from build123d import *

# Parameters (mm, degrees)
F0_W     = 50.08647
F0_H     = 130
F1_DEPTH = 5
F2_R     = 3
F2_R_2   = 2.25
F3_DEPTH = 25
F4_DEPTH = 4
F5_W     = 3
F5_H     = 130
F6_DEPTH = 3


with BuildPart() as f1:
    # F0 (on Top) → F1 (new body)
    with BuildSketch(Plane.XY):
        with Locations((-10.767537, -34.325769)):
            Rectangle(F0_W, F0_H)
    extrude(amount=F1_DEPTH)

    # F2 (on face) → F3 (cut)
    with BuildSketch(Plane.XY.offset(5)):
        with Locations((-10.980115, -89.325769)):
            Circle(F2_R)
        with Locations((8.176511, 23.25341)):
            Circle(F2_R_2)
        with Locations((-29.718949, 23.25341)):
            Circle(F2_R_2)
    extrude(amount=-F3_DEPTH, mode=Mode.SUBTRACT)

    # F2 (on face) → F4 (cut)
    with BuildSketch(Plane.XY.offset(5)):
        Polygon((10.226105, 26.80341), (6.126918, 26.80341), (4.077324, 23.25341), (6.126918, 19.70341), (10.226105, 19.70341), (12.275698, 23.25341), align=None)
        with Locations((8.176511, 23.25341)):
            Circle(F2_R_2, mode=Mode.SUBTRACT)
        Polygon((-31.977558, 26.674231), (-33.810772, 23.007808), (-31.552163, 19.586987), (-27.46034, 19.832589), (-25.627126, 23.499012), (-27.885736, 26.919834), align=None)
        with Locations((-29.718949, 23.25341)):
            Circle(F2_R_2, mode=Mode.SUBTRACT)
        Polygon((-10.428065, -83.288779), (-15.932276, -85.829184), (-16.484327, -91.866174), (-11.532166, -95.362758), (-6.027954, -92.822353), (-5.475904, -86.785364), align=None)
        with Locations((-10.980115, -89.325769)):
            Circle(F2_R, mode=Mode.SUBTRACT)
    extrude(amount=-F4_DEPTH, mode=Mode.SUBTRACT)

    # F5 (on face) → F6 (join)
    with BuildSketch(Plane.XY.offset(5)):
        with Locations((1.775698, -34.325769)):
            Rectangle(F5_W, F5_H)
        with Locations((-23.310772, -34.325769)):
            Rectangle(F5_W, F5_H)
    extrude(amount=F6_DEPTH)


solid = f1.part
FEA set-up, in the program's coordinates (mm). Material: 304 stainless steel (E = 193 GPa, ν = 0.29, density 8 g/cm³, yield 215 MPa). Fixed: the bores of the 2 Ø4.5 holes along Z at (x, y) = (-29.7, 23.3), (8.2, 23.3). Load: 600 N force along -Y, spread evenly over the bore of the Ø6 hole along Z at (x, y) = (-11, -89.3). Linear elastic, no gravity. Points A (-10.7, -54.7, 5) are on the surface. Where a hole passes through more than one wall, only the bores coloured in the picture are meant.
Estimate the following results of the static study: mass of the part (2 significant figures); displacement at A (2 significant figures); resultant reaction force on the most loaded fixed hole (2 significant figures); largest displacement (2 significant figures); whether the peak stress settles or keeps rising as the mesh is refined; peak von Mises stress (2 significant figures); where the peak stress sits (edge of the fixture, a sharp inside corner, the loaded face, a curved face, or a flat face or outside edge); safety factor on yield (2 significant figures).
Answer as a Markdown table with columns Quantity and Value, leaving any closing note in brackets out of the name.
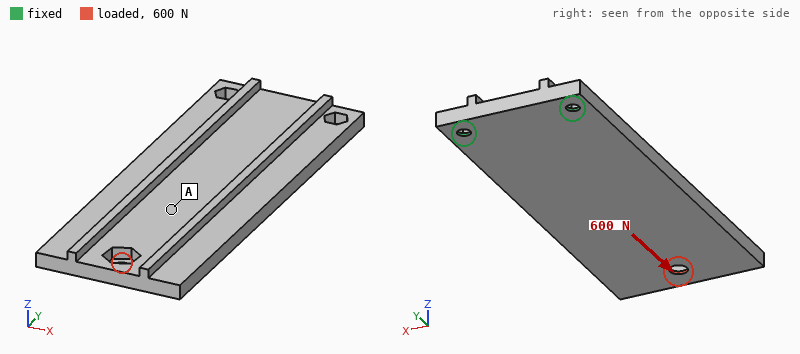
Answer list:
| Quantity | Value |
|---|---|
| mass of the part | 270 g |
| displacement at A | 23 µm |
| resultant reaction force on the most loaded fixed hole | 300 N |
| largest displacement | 61 µm |
| whether the peak stress settles or keeps rising as the mesh is refined | settles |
| peak von Mises stress | 60 MPa |
| where the peak stress sits | the loaded face |
| safety factor on yield | 3.6 |
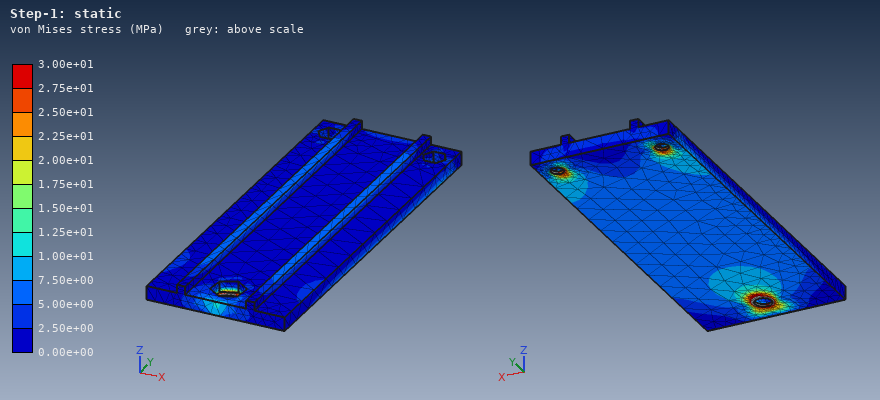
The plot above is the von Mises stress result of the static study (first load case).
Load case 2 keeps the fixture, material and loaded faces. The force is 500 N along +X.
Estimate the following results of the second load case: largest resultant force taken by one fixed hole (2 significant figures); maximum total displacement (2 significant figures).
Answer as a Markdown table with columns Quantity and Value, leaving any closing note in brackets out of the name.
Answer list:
| Quantity | Value |
|---|---|
| largest resultant force taken by one fixed hole | 1.5 kN |
| maximum total displacement | 60 µm |
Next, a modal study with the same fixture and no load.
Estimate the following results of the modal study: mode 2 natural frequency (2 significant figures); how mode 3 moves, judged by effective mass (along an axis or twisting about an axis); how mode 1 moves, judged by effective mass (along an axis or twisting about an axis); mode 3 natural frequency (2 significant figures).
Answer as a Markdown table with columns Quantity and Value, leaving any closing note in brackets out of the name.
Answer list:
| Quantity | Value |
|---|---|
| mode 2 natural frequency | 1300 Hz |
| how mode 3 moves, judged by effective mass | along Z |
| how mode 1 moves, judged by effective mass | along Z |
| mode 3 natural frequency | 1500 Hz |
